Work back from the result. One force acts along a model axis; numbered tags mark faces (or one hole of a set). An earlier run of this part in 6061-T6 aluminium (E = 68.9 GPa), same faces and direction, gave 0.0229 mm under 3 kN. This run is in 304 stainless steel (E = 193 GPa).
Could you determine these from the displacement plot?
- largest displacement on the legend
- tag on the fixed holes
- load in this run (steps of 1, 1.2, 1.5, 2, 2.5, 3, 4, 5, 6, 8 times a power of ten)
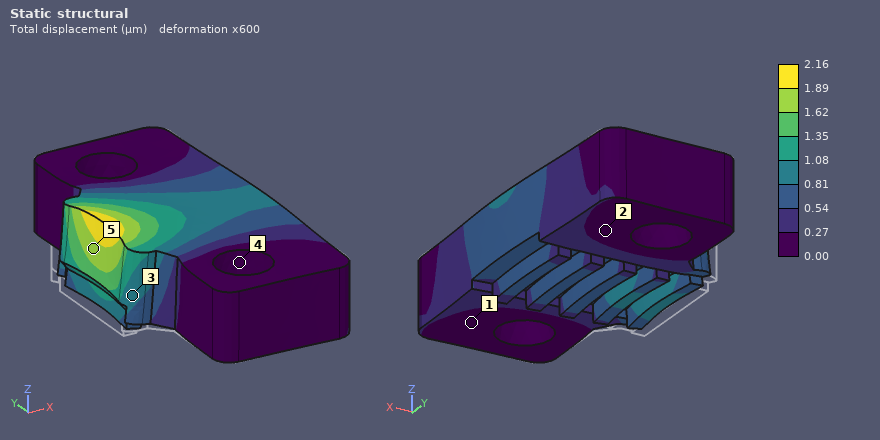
2.16 µm
4
800 N
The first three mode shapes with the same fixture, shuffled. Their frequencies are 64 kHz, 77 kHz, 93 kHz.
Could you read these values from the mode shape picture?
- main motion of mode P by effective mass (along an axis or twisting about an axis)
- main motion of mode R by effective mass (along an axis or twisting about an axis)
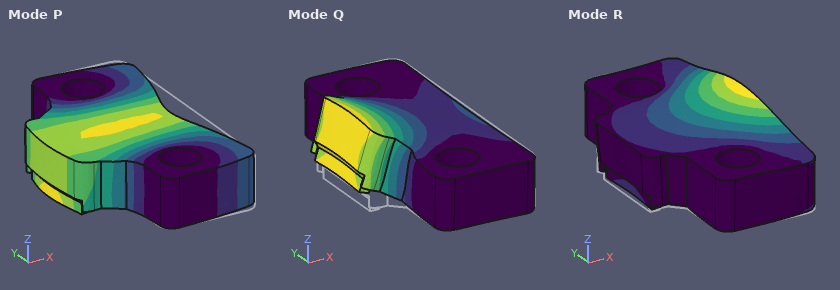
along X
along Z
